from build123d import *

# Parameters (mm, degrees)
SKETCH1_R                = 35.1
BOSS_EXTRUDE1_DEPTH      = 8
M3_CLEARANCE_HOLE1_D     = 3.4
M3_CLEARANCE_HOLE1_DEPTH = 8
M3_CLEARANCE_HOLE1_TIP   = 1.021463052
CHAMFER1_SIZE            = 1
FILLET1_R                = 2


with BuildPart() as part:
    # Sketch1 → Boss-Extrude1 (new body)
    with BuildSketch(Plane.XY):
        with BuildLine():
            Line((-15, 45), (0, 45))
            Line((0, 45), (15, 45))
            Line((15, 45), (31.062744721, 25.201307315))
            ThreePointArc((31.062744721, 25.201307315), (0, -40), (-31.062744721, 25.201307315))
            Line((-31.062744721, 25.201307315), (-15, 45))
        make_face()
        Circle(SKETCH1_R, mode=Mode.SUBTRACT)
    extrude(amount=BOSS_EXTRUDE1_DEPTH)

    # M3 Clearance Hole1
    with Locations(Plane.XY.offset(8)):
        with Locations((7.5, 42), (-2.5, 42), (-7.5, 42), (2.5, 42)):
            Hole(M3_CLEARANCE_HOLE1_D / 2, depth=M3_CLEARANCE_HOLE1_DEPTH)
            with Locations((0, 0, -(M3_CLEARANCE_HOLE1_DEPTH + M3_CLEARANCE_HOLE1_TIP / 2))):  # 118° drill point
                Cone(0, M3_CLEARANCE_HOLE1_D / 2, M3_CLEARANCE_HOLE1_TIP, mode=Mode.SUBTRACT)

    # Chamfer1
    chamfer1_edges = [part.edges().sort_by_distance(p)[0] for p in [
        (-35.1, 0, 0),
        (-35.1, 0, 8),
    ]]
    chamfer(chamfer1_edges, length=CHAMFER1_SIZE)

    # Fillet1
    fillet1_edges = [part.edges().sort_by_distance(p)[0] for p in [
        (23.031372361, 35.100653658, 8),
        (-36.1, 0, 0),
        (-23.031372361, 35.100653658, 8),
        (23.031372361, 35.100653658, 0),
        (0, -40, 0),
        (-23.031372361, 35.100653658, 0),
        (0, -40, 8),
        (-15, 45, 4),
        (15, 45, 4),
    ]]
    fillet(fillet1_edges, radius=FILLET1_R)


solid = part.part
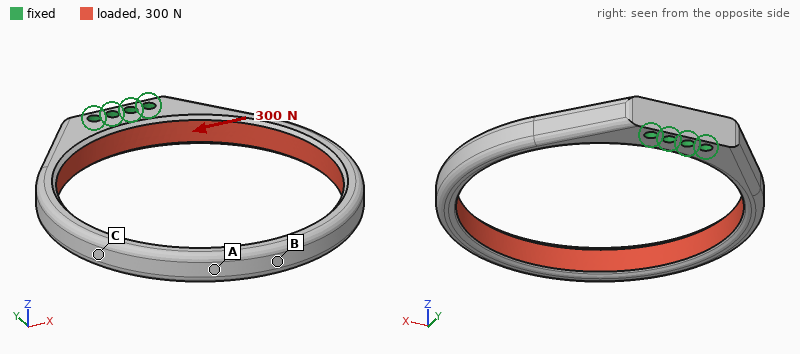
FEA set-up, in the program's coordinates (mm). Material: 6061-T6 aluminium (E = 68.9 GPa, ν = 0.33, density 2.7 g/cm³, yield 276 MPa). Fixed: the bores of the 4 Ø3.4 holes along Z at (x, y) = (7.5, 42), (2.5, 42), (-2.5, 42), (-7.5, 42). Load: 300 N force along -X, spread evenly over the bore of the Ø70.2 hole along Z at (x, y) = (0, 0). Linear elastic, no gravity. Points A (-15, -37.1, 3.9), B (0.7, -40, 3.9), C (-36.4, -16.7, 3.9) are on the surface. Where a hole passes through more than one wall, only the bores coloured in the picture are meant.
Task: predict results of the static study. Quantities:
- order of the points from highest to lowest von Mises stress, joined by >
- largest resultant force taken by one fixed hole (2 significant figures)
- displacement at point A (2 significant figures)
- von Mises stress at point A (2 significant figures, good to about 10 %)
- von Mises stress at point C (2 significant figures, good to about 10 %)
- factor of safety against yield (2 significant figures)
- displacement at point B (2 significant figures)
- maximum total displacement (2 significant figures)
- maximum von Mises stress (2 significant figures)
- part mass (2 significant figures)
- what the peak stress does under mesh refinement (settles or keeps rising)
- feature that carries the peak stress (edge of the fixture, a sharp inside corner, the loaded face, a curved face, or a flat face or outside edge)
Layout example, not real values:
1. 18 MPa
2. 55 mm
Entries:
1. C > A > B
2. 570 N
3. 0.61 mm
4. 27 MPa
5. 41 MPa
6. 2.9
7. 0.61 mm
8. 0.61 mm
9. 94 MPa
10. 28 g
11. settles
12. the loaded face
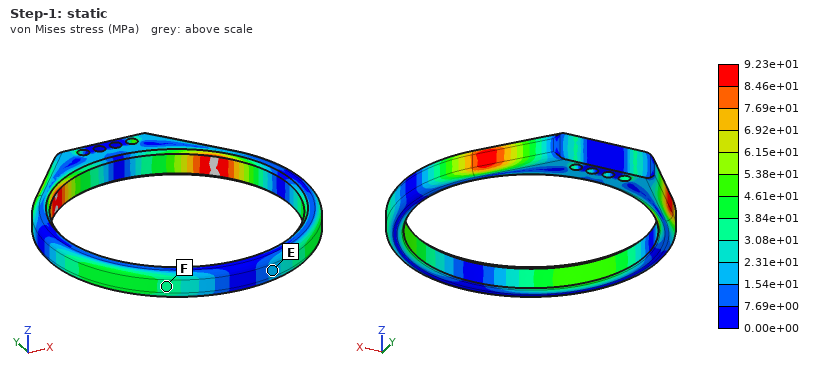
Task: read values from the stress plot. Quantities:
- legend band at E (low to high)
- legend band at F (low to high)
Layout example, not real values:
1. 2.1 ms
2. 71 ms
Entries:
1. 1.54e+01 to 2.31e+01 MPa
2. 3.08e+01 to 3.84e+01 MPa
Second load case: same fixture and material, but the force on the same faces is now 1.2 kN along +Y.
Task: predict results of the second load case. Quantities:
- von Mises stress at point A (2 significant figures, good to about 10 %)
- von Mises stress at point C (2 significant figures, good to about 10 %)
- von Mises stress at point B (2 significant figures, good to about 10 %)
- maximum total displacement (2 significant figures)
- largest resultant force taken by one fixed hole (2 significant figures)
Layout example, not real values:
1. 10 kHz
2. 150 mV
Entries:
1. 52 MPa
2. 44 MPa
3. 70 MPa
4. 0.35 mm
5. 1.5 kN
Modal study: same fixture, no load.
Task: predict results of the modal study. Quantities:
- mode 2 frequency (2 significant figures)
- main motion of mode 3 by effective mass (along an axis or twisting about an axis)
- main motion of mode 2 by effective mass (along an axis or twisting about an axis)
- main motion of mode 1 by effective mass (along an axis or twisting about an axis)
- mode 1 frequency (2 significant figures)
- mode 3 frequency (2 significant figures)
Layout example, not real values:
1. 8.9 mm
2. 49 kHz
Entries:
1. 790 Hz
2. twisting about Y
3. along X
4. along Z
5. 610 Hz
6. 1500 Hz
